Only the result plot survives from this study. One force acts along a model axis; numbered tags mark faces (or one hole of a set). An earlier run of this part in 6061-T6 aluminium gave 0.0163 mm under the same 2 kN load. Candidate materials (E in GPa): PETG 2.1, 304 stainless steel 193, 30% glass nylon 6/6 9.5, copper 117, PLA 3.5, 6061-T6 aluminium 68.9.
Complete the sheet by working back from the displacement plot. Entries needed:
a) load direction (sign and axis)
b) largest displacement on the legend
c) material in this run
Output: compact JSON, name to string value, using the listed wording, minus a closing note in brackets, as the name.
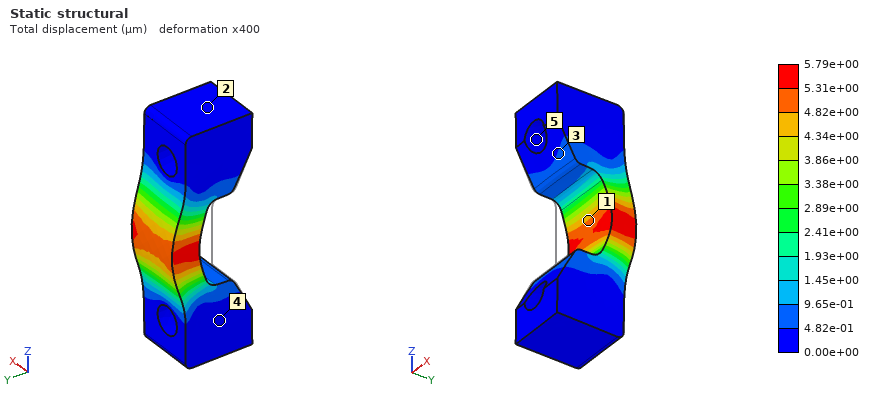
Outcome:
{"load direction": "+Y", "largest displacement on the legend": "5.79e+00 µm", "material in this run": "304 stainless steel"}
